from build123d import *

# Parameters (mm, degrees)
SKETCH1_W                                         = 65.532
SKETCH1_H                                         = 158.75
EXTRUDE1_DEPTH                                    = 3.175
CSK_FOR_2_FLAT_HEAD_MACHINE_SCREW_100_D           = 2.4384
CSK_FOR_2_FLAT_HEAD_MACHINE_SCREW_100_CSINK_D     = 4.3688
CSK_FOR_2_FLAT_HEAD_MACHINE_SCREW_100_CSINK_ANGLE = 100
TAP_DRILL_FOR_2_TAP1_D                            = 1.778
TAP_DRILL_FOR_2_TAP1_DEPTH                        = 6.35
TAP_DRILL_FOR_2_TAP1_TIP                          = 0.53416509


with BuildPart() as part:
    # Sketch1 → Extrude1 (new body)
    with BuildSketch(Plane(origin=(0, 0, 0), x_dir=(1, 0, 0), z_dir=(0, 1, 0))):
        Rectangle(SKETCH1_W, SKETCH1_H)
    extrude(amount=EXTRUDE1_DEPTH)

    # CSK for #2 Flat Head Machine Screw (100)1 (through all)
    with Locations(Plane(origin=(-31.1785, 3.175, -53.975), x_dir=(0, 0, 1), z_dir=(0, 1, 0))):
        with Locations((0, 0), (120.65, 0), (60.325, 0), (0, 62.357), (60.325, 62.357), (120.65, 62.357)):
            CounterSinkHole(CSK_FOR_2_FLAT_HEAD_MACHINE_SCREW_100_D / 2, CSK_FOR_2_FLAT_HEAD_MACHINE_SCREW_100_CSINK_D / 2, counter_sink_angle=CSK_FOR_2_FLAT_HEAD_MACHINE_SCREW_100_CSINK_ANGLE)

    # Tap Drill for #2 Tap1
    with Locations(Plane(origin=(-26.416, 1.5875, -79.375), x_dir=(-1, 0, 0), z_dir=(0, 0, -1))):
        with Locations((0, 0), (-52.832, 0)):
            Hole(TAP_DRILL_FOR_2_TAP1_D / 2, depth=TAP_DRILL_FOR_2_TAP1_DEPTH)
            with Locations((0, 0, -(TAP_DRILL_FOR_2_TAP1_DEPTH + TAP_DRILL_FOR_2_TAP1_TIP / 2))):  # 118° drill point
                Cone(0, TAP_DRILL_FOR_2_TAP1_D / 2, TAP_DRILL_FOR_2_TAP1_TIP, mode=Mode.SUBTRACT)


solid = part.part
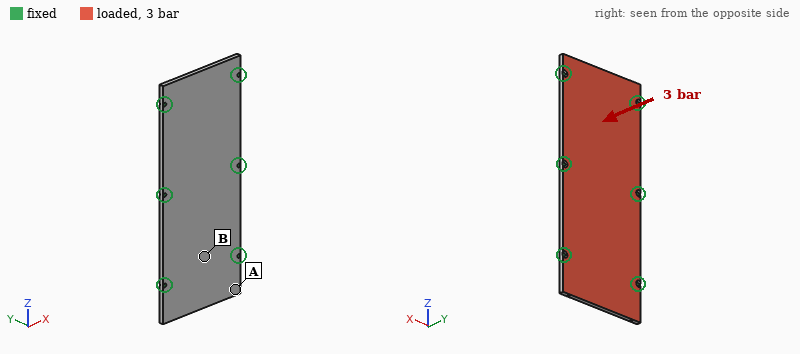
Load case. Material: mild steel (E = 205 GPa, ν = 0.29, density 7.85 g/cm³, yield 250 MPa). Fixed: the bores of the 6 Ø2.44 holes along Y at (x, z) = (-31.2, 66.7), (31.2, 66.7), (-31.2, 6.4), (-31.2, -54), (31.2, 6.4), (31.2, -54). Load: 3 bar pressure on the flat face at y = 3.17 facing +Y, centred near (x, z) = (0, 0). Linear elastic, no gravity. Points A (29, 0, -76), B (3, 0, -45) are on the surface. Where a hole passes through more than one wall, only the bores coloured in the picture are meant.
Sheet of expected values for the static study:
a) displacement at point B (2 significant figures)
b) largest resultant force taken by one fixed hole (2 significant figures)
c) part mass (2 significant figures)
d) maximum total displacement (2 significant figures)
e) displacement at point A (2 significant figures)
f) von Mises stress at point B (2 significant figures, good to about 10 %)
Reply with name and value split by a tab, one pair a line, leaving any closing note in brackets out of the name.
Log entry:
displacement at point B	57 µm
largest resultant force taken by one fixed hole	640 N
part mass	260 g
maximum total displacement	94 µm
displacement at point A	41 µm
von Mises stress at point B	48 MPa
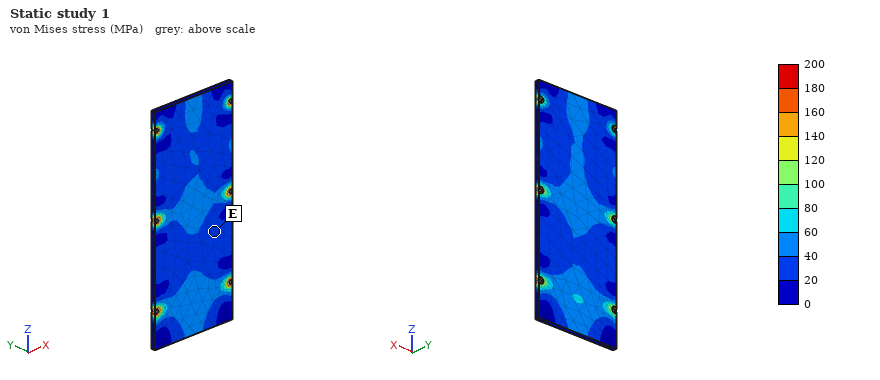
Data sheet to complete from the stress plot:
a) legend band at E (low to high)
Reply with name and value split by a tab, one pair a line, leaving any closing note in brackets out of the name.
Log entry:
legend band at E	20 to 40 MPa
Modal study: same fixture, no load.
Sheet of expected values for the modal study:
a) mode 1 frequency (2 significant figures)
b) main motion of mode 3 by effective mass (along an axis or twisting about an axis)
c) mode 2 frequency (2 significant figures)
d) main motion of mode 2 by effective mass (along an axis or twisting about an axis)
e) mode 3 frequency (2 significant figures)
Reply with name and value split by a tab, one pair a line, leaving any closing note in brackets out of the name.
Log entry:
mode 1 frequency	2200 Hz
main motion of mode 3 by effective mass	twisting about X
mode 2 frequency	2500 Hz
main motion of mode 2 by effective mass	along Y
mode 3 frequency	2600 Hz
